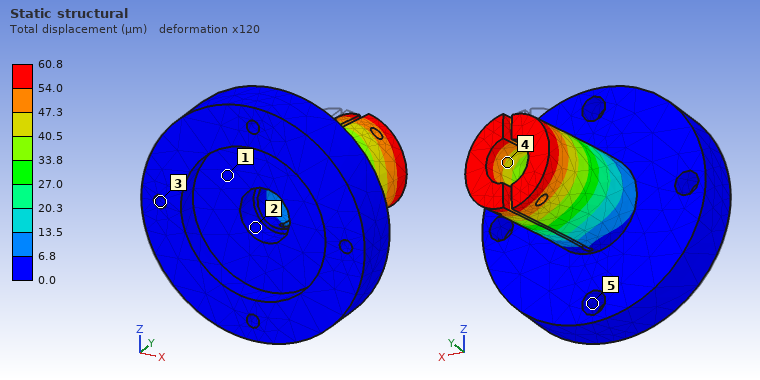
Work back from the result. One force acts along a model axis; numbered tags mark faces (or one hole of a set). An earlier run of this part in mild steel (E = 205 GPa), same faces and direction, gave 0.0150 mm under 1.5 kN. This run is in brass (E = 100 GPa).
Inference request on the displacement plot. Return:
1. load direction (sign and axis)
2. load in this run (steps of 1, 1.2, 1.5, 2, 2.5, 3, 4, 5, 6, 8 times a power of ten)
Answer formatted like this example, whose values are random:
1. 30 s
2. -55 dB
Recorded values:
1. +X
2. 3 kN
